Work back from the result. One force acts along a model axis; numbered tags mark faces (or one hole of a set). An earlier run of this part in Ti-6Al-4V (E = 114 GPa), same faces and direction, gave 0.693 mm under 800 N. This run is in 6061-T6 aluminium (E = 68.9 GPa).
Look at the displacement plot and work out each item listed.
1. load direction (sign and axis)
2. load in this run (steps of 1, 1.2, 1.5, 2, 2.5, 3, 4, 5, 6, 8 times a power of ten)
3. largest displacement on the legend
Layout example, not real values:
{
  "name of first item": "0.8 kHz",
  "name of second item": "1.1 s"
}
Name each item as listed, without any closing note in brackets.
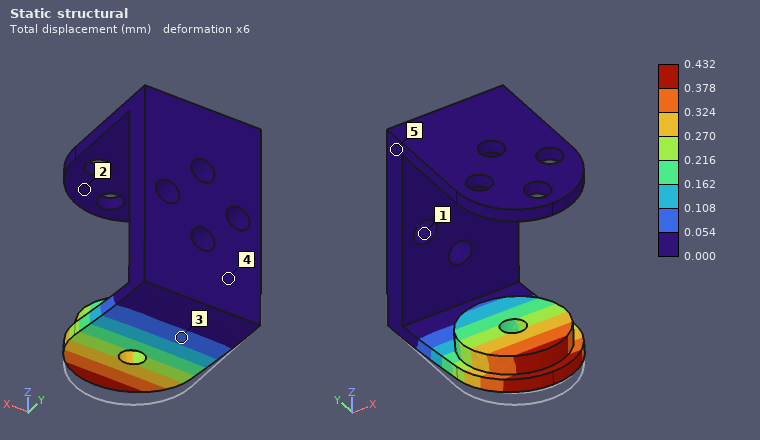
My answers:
{
  "load direction": "+Z",
  "load in this run": "300 N",
  "largest displacement on the legend": "0.432 mm"
}
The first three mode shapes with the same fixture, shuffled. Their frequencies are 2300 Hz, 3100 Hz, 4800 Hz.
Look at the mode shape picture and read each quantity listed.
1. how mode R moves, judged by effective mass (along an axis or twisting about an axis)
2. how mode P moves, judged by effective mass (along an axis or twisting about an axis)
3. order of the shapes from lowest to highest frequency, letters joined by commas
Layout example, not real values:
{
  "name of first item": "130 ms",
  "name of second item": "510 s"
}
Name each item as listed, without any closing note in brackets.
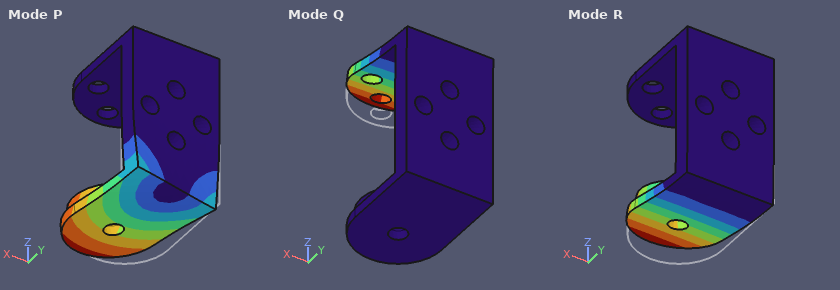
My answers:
{
  "how mode R moves, judged by effective mass": "along Z",
  "how mode P moves, judged by effective mass": "along X",
  "order of the shapes from lowest to highest frequency, letters joined by commas": "R, Q, P"
}
